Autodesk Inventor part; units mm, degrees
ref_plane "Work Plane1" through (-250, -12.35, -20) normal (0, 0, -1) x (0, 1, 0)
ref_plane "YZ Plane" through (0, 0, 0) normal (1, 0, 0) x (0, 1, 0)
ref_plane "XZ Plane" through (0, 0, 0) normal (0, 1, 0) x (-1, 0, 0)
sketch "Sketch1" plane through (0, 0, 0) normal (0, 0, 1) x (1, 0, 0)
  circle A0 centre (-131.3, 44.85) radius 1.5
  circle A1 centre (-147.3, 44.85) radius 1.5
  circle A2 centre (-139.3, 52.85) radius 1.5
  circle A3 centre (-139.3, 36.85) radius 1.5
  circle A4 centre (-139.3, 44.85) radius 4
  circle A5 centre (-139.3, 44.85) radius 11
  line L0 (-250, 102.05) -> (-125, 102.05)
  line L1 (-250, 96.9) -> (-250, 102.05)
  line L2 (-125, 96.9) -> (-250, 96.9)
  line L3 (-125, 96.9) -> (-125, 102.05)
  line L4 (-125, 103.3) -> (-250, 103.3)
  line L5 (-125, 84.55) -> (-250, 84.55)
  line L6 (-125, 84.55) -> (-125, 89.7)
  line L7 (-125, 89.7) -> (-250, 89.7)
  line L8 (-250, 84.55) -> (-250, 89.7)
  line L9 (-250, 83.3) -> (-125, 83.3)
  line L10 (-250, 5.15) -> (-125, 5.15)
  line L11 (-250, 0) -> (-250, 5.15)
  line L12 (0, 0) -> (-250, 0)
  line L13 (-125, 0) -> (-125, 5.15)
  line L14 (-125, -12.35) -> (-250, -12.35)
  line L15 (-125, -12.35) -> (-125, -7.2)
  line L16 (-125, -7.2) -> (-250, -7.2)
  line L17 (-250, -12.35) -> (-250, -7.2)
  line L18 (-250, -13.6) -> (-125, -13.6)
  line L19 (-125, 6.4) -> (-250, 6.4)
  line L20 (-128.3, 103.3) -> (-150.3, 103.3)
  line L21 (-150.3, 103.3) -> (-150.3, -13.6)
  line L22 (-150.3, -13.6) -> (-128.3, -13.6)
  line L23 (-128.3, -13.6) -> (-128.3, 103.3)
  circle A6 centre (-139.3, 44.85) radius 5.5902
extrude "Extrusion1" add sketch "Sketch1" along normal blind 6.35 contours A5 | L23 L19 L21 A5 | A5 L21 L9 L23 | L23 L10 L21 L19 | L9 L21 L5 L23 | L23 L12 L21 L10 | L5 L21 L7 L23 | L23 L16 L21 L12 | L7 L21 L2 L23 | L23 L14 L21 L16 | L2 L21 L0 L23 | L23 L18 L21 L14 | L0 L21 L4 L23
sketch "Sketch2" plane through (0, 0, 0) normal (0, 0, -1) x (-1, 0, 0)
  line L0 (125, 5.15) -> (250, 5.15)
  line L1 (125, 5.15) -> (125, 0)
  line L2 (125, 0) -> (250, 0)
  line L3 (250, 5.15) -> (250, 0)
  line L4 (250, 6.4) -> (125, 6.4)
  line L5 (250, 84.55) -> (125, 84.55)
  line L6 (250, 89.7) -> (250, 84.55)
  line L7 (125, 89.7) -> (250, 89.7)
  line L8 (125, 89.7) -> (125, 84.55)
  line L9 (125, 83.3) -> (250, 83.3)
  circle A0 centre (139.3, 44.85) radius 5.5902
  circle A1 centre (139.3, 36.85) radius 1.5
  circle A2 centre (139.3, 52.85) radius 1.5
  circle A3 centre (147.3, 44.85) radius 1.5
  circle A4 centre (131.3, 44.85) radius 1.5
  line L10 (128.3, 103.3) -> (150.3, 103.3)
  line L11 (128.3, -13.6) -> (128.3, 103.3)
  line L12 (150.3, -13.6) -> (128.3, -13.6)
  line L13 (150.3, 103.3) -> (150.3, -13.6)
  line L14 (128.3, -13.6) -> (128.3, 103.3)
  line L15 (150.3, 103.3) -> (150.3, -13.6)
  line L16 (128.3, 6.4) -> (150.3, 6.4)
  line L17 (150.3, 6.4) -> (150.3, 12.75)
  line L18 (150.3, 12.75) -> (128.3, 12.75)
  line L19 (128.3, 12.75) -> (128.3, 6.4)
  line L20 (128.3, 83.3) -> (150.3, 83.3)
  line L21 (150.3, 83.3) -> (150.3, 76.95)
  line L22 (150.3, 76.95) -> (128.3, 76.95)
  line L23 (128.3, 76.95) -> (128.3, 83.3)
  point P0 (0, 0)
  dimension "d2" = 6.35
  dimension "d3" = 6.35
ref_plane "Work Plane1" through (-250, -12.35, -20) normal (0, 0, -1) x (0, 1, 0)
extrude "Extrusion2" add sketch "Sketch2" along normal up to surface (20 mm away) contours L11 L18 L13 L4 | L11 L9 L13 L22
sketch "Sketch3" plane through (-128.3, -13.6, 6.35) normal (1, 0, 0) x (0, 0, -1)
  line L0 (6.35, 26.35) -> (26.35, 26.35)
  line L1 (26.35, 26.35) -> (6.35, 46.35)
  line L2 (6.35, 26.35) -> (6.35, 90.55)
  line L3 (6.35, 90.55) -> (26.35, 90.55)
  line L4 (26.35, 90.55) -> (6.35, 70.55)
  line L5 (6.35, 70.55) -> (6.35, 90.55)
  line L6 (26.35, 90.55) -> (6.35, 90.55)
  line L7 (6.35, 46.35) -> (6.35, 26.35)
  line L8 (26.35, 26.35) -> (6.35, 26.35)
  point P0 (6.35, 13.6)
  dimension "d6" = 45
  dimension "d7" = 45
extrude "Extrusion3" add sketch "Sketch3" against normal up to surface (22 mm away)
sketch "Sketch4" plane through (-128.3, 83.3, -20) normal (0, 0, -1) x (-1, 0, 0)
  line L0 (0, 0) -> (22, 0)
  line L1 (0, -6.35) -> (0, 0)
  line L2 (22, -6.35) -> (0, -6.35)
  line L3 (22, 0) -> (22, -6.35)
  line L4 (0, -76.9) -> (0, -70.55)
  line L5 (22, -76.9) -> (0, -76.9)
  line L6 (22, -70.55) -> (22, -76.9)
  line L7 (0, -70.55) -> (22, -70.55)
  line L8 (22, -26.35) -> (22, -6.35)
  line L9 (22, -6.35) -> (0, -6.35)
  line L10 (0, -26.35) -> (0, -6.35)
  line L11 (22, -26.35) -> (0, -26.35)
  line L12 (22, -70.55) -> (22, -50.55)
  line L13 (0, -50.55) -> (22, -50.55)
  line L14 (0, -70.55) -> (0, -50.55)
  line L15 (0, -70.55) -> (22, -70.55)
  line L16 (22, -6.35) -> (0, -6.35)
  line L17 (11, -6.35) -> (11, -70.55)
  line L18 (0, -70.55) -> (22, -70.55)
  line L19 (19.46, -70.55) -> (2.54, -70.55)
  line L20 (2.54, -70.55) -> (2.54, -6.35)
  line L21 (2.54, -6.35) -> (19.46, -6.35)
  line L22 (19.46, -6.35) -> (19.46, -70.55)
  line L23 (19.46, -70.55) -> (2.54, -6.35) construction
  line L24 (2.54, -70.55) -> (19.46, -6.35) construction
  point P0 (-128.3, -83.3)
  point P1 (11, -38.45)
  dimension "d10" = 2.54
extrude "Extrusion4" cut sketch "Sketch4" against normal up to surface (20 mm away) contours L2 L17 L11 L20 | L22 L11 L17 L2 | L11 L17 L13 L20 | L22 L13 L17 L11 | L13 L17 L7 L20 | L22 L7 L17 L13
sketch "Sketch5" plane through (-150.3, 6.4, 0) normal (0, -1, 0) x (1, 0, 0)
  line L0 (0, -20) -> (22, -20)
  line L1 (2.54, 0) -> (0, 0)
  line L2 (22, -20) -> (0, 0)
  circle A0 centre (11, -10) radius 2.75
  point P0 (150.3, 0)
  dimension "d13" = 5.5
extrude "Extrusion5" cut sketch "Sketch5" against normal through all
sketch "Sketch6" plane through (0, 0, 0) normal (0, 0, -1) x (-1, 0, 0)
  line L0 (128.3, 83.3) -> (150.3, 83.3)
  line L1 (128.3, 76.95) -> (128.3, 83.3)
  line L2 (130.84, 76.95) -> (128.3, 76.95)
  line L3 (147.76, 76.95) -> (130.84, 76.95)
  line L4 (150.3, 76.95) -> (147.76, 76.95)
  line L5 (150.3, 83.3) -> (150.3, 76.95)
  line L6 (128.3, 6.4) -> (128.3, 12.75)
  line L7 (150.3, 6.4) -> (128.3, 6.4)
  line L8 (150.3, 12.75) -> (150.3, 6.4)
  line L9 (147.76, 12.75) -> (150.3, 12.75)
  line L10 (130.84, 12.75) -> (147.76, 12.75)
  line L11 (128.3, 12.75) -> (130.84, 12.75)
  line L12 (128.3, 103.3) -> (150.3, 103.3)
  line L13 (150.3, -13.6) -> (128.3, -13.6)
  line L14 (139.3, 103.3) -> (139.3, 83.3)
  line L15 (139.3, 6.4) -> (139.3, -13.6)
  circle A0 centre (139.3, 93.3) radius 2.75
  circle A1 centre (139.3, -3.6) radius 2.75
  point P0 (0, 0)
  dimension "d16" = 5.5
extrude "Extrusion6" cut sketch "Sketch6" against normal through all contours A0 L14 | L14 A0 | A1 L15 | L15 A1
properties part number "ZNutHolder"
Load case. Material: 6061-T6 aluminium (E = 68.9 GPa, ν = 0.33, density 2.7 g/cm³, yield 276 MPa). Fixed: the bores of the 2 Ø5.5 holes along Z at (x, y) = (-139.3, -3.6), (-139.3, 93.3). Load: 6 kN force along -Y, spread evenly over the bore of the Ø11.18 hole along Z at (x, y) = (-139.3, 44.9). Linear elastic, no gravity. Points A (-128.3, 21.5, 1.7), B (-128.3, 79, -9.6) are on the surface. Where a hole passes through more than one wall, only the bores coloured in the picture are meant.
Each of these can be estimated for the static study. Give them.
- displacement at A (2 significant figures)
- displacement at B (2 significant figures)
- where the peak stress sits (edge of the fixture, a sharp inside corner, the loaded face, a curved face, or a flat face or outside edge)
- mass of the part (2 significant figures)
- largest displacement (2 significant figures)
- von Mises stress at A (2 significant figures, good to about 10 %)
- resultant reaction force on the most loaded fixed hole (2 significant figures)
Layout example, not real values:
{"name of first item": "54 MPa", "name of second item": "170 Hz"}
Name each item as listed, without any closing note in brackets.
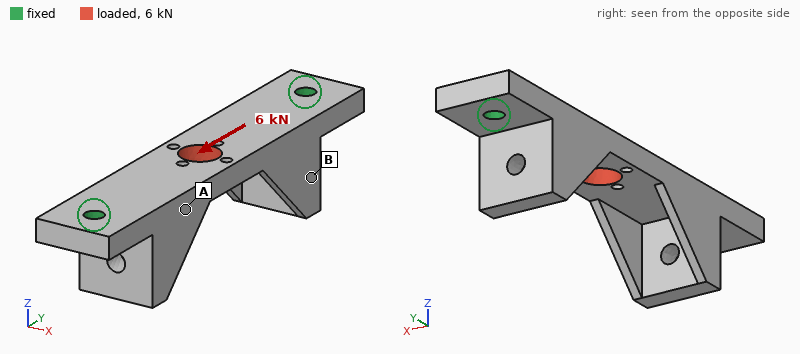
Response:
{"displacement at A": "9.2 µm", "displacement at B": "8.6 µm", "where the peak stress sits": "a curved face", "mass of the part": "61 g", "largest displacement": "18 µm", "von Mises stress at A": "17 MPa", "resultant reaction force on the most loaded fixed hole": "3.0 kN"}
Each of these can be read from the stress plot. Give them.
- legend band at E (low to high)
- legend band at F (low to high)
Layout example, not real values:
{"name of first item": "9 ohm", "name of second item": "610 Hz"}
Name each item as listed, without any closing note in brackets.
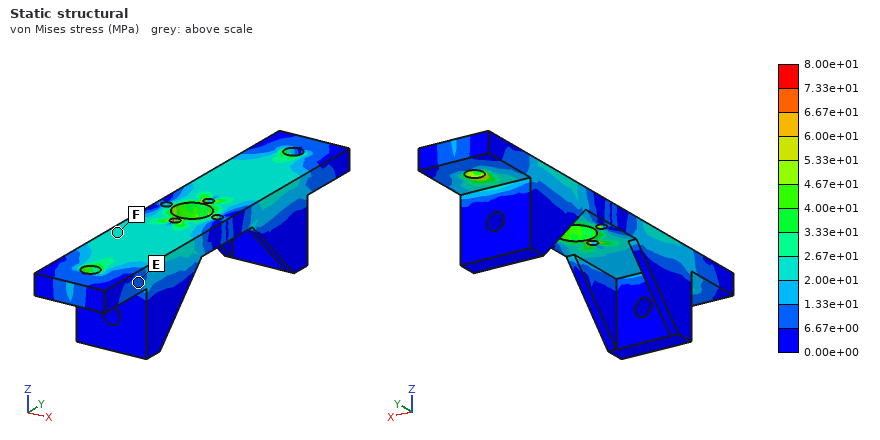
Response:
{"legend band at E": "6.67e+00 to 1.33e+01 MPa", "legend band at F": "2.00e+01 to 2.67e+01 MPa"}
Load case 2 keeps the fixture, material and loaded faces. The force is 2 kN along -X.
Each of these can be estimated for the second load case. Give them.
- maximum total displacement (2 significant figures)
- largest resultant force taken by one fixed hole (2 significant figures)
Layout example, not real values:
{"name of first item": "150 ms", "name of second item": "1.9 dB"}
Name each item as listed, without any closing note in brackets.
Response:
{"maximum total displacement": "68 µm", "largest resultant force taken by one fixed hole": "1.0 kN"}
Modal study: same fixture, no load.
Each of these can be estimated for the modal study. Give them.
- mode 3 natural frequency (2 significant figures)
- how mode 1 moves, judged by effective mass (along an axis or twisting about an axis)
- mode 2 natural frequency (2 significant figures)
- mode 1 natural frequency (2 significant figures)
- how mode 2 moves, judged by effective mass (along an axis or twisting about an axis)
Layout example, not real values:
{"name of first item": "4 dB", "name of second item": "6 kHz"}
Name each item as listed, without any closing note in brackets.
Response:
{"mode 3 natural frequency": "6900 Hz", "how mode 1 moves, judged by effective mass": "along Z", "mode 2 natural frequency": "5500 Hz", "mode 1 natural frequency": "3000 Hz", "how mode 2 moves, judged by effective mass": "along X"}
